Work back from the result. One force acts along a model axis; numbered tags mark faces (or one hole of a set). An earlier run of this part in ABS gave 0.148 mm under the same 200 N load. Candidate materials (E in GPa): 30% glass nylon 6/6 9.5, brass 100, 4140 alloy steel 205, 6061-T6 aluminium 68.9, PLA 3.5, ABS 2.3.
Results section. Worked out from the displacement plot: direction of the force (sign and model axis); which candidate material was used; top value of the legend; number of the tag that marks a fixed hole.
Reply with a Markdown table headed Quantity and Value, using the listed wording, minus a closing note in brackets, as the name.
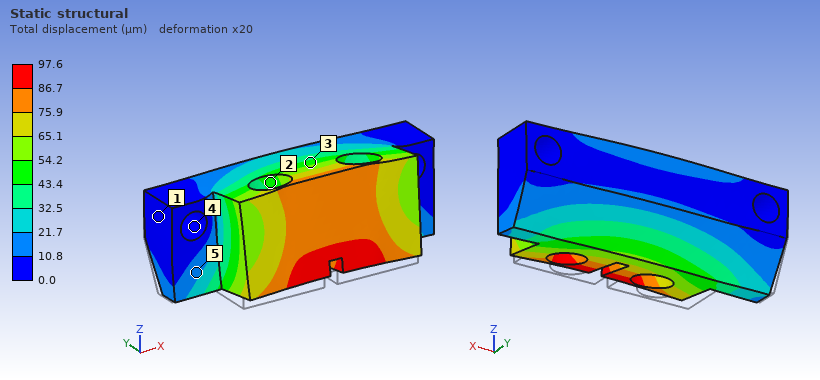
| Quantity | Value |
|---|---|
| direction of the force | +Z |
| which candidate material was used | PLA |
| top value of the legend | 97.6 µm |
| number of the tag that marks a fixed hole | 4 |
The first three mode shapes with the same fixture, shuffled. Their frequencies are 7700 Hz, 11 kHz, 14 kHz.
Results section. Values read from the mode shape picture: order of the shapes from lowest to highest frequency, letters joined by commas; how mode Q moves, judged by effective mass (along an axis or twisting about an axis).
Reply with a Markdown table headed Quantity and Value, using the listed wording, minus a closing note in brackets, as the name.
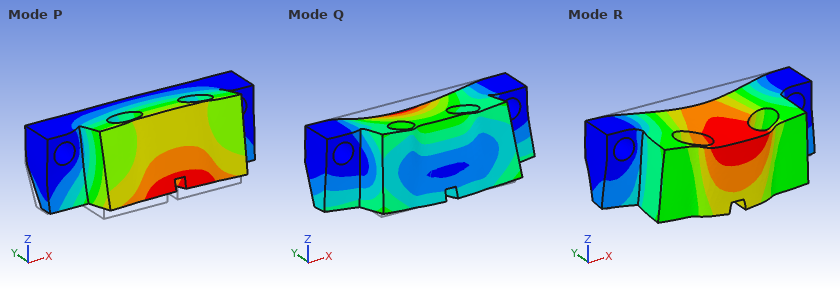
| Quantity | Value |
|---|---|
| order of the shapes from lowest to highest frequency, letters joined by commas | P, R, Q |
| how mode Q moves, judged by effective mass | along Z |
